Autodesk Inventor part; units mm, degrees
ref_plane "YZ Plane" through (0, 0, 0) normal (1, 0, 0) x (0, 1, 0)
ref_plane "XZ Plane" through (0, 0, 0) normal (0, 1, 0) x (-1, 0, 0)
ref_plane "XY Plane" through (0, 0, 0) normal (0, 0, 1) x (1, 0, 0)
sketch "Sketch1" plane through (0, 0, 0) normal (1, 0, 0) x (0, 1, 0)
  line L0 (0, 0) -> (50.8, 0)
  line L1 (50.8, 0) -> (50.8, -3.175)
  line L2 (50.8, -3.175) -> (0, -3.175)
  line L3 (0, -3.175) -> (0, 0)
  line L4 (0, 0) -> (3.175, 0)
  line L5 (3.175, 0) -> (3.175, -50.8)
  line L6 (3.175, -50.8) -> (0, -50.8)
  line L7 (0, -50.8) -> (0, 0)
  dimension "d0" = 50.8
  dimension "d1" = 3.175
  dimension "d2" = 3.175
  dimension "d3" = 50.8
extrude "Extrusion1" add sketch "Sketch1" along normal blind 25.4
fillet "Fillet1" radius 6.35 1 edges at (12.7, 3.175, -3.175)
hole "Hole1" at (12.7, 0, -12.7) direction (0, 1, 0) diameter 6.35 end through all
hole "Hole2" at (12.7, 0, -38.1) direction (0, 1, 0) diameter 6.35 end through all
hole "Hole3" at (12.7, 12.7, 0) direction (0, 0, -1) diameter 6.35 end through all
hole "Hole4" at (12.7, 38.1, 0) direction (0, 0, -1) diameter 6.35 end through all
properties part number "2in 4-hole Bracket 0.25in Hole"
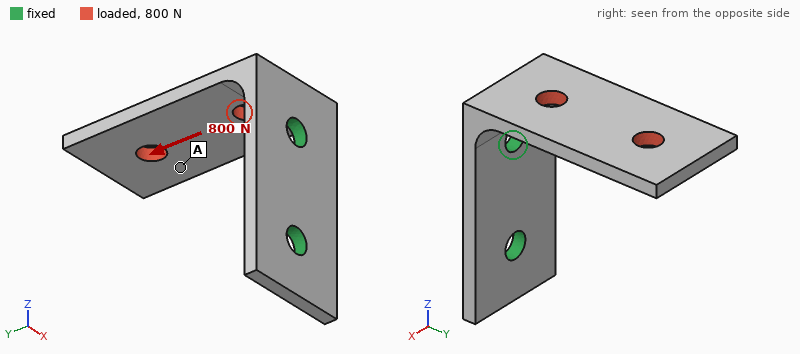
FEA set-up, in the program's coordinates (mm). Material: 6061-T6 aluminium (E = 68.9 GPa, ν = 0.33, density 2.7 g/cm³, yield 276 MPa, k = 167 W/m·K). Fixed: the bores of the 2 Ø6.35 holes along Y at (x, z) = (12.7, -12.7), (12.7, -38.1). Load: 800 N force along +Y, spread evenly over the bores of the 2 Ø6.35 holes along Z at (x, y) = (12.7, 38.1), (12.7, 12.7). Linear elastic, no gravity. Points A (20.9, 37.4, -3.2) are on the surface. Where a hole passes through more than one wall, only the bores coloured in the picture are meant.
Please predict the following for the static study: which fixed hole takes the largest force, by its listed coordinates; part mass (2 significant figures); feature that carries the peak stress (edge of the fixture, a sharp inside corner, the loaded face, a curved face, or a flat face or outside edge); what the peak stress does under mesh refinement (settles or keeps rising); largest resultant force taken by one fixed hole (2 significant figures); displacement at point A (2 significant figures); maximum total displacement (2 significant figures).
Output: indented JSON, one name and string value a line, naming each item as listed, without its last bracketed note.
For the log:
{
  "which fixed hole takes the largest force, by its listed coordinates": "(12.7, -12.7)",
  "part mass": "21 g",
  "feature that carries the peak stress": "edge of the fixture",
  "what the peak stress does under mesh refinement": "keeps rising",
  "largest resultant force taken by one fixed hole": "840 N",
  "displacement at point A": "0.24 mm",
  "maximum total displacement": "0.33 mm"
}
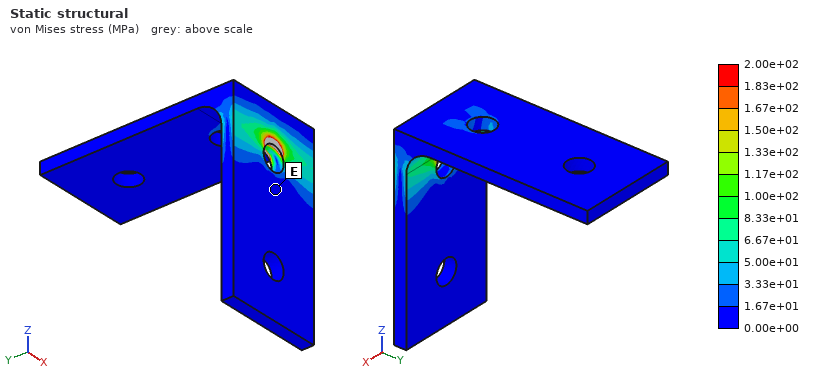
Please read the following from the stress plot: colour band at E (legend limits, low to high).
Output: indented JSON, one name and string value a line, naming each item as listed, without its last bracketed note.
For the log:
{
  "colour band at E": "0.00e+00 to 1.67e+01 MPa"
}
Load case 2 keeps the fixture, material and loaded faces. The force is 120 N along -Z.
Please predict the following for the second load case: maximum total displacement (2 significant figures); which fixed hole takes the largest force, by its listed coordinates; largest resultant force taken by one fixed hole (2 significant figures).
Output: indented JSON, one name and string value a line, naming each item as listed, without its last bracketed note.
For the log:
{
  "maximum total displacement": "0.44 mm",
  "which fixed hole takes the largest force, by its listed coordinates": "(12.7, -12.7)",
  "largest resultant force taken by one fixed hole": "120 N"
}
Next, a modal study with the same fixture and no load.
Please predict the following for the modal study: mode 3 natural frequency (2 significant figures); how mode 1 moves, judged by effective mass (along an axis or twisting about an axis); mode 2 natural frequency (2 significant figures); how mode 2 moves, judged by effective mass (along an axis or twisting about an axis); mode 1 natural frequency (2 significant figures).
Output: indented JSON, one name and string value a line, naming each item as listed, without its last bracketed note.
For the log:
{
  "mode 3 natural frequency": "4400 Hz",
  "how mode 1 moves, judged by effective mass": "along Z",
  "mode 2 natural frequency": "2000 Hz",
  "how mode 2 moves, judged by effective mass": "along X",
  "mode 1 natural frequency": "980 Hz"
}
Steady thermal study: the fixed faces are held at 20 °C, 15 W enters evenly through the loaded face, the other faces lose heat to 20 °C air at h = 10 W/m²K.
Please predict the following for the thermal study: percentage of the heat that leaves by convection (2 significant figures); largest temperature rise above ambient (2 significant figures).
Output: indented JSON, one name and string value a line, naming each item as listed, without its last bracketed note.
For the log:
{
  "percentage of the heat that leaves by convection": "5.0 %",
  "largest temperature rise above ambient": "36 K"
}
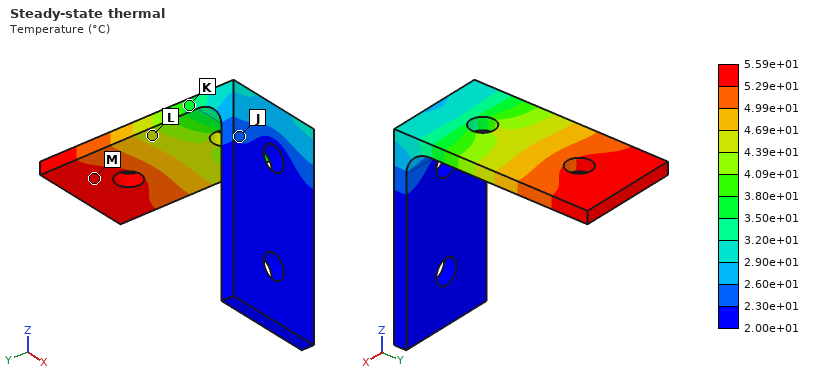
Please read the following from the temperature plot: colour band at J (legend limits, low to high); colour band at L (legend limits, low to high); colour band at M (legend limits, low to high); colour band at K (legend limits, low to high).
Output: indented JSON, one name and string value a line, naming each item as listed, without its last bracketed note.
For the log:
{
  "colour band at J": "2.30e+01 to 2.60e+01 °C",
  "colour band at L": "4.39e+01 to 4.69e+01 °C",
  "colour band at M": "5.29e+01 to 5.59e+01 °C",
  "colour band at K": "3.50e+01 to 3.80e+01 °C"
}
